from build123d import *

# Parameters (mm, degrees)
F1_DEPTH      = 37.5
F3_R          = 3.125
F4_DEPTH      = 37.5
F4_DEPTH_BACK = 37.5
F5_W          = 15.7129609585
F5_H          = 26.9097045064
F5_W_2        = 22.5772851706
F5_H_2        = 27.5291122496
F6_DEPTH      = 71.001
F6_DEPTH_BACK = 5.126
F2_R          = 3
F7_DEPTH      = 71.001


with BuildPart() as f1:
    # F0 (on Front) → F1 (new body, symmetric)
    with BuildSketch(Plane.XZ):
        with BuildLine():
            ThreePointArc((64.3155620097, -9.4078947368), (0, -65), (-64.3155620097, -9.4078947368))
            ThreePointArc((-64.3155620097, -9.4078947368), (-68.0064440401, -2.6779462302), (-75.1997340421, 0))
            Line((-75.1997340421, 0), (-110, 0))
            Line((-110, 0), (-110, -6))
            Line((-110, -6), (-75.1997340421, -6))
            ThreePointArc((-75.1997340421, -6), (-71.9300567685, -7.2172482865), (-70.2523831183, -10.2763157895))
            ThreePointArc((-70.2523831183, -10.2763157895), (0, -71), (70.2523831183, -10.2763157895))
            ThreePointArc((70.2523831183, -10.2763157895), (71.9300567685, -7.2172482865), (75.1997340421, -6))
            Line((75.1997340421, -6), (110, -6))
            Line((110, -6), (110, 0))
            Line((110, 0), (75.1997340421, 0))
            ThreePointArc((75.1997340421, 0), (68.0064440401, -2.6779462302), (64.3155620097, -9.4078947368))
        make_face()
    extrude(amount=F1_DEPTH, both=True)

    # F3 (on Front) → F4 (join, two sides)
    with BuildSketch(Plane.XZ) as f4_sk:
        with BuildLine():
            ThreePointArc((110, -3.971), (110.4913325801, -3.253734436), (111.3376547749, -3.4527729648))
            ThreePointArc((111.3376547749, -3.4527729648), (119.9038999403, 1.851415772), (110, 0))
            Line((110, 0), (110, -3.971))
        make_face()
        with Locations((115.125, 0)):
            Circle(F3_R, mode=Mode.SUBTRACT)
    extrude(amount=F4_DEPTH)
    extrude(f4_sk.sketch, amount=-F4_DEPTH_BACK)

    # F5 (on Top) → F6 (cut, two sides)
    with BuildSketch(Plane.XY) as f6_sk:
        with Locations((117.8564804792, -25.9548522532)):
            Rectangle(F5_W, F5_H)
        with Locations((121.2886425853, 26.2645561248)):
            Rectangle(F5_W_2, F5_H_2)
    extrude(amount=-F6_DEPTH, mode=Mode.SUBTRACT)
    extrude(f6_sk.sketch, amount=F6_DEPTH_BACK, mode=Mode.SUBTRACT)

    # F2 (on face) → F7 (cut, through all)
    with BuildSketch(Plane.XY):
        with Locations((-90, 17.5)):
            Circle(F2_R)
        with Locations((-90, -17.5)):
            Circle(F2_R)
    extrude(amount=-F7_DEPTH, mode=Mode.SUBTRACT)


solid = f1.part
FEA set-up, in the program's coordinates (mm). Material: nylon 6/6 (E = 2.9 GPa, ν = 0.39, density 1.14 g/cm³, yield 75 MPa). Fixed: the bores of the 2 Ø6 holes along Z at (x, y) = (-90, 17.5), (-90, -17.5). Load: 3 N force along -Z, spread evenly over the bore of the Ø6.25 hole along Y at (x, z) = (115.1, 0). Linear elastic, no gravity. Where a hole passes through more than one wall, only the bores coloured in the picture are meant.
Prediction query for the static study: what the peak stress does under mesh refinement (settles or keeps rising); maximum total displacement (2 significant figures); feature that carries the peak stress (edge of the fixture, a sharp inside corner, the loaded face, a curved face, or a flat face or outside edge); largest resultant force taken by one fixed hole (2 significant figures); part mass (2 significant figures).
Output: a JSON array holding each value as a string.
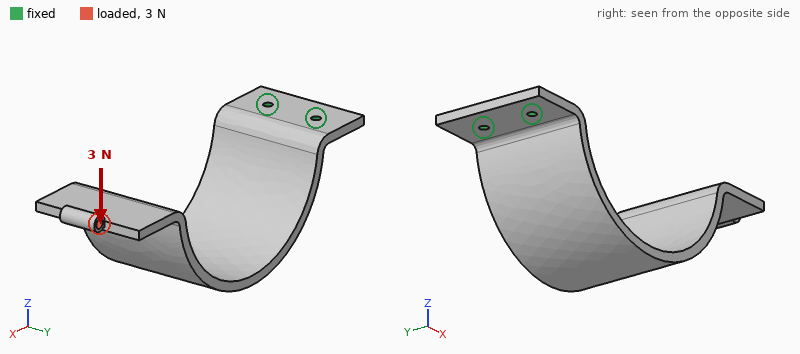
["keeps rising", "3.0 mm", "edge of the fixture", "1.7 N", "150 g"]
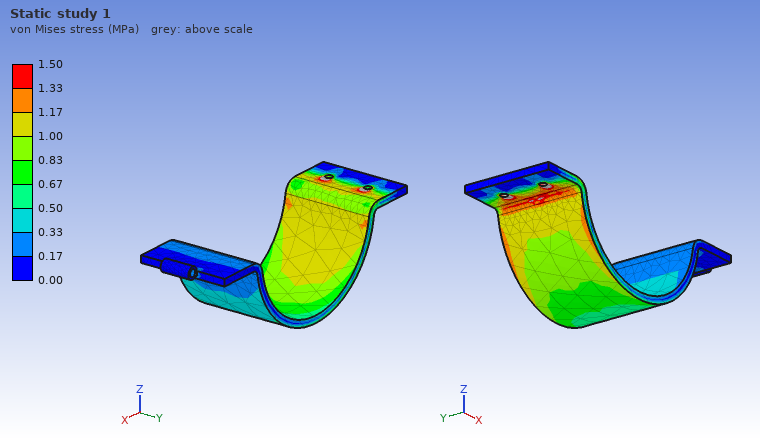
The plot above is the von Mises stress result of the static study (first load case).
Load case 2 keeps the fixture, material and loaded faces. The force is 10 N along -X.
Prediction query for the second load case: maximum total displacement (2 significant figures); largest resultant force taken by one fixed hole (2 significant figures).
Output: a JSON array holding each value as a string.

["2.9 mm", "5.0 N"]
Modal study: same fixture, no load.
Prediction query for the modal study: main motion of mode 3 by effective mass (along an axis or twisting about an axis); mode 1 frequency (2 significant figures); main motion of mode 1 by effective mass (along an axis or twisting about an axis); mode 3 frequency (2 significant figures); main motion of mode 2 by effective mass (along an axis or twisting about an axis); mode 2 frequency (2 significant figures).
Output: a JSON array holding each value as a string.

["along X", "28 Hz", "along Z", "89 Hz", "along Y", "48 Hz"]
